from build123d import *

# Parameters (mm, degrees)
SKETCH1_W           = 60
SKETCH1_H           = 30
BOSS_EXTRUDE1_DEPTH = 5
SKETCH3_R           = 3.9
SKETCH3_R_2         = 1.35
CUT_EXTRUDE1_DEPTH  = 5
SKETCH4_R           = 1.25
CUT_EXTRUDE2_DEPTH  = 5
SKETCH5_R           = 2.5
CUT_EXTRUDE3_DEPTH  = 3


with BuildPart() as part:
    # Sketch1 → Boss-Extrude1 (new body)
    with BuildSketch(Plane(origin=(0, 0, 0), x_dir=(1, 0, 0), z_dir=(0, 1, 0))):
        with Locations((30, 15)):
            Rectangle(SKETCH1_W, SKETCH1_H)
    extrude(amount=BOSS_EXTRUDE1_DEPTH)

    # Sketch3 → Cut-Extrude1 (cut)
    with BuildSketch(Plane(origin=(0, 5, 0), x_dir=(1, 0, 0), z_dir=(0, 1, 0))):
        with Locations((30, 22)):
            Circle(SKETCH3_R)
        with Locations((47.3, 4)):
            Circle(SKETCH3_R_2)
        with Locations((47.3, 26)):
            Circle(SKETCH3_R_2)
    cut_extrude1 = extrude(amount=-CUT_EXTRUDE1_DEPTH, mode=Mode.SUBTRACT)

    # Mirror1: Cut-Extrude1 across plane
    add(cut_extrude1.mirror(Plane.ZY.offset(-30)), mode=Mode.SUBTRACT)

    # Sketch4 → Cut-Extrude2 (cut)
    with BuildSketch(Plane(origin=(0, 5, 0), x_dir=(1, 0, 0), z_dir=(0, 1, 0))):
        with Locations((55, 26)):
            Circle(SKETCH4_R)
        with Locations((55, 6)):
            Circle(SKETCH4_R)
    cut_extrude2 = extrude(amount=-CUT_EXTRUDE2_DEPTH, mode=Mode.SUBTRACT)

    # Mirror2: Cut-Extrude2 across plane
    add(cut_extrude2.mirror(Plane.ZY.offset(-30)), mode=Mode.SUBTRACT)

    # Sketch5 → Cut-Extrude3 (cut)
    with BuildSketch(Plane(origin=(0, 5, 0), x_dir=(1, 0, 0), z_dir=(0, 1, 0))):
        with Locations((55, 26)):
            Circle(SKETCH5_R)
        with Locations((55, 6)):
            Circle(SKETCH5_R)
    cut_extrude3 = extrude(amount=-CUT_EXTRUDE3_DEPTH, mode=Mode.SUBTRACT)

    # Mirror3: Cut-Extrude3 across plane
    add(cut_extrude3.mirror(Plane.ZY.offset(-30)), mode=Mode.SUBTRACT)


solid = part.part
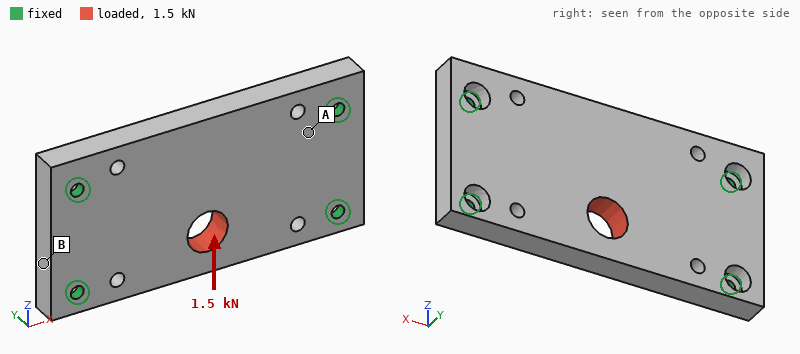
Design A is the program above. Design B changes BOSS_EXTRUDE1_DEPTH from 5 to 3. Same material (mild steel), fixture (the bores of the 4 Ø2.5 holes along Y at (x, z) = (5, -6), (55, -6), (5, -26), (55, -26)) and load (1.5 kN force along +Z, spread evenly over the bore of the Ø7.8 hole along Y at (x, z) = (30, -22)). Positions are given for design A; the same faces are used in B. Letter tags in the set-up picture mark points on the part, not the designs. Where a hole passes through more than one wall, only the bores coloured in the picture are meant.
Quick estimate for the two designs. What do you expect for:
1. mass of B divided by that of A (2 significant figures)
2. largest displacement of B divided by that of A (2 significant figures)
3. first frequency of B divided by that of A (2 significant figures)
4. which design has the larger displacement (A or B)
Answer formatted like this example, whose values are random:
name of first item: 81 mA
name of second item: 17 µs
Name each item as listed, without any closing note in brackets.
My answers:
mass of B divided by that of A: 0.61
largest displacement of B divided by that of A: 1.5
first frequency of B divided by that of A: 0.75
which design has the larger displacement: B
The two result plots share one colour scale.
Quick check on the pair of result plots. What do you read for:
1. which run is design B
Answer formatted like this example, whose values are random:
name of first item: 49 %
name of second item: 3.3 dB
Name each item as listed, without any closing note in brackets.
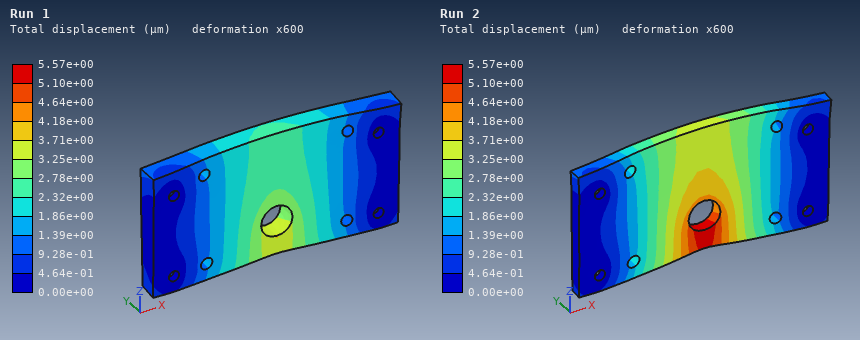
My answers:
which run is design B: Run 2
